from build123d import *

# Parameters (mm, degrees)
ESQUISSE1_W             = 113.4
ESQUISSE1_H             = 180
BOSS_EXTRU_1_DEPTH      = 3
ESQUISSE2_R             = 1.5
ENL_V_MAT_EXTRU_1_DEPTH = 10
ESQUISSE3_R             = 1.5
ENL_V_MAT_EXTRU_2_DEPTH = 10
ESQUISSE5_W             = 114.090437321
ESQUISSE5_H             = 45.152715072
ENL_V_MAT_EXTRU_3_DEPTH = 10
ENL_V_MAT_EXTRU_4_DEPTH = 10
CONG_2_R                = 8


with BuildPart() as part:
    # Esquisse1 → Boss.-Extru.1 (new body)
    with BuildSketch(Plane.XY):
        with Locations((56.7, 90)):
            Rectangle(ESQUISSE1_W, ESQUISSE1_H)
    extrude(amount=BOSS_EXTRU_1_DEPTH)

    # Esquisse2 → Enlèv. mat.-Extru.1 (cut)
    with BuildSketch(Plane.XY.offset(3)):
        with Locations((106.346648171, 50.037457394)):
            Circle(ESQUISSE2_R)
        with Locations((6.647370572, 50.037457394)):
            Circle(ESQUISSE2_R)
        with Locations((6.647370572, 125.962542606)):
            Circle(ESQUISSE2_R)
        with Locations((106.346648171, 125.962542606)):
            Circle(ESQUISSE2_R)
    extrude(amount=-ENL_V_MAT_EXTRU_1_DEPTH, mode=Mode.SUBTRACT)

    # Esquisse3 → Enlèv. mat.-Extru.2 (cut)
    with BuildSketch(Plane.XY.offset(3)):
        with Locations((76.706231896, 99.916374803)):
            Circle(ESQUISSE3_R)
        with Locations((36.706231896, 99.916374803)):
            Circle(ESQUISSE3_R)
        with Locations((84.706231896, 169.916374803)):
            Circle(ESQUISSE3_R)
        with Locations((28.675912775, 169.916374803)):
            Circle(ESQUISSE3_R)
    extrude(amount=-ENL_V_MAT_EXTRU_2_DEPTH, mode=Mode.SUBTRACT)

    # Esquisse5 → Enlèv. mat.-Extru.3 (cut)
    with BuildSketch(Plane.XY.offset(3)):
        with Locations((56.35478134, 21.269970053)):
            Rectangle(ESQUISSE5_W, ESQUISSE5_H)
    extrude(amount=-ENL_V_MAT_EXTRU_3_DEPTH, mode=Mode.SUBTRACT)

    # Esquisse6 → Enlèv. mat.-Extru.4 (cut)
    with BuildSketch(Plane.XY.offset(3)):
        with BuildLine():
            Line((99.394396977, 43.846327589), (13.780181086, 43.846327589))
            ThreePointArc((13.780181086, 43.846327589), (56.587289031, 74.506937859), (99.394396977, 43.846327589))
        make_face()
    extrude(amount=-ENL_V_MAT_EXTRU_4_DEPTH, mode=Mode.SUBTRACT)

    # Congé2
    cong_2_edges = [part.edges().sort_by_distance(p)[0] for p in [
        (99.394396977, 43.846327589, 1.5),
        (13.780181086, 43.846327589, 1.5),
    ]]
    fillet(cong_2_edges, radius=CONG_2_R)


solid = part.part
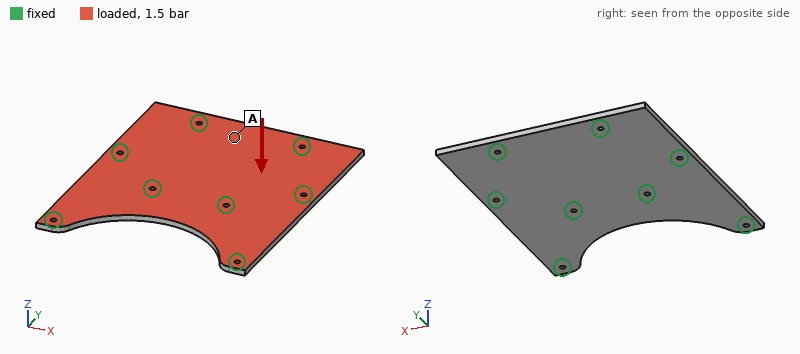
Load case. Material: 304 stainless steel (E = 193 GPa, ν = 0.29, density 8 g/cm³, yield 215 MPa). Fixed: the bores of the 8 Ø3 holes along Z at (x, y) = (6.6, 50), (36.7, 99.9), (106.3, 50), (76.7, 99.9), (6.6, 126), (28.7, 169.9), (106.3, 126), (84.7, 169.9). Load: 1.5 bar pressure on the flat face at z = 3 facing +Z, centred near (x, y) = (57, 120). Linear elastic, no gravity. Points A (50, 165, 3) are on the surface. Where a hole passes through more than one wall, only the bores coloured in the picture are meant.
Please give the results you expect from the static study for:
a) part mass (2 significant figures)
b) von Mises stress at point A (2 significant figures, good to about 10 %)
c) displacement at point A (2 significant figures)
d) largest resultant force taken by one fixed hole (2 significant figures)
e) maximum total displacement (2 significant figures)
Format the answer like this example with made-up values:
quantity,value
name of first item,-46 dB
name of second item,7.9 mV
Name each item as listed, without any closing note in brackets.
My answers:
quantity,value
part mass,320 g
von Mises stress at point A,13 MPa
displacement at point A,14 µm
largest resultant force taken by one fixed hole,360 N
maximum total displacement,24 µm
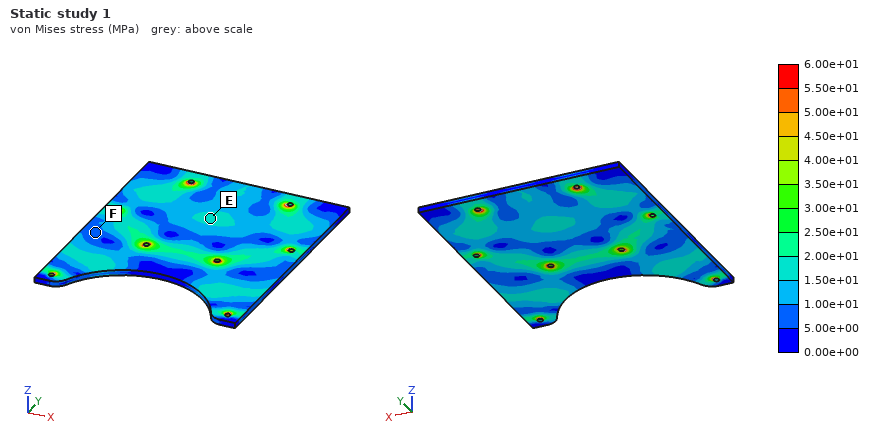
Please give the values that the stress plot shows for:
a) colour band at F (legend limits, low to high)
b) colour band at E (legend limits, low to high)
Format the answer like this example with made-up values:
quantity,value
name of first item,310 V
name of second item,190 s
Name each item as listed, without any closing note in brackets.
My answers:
quantity,value
colour band at F,5.00e+00 to 1.00e+01 MPa
colour band at E,1.50e+01 to 2.00e+01 MPa
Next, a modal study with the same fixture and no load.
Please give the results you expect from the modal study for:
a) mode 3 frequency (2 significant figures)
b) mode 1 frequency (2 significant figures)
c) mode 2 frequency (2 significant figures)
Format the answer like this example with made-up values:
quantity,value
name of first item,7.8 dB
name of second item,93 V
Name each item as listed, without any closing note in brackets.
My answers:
quantity,value
mode 3 frequency,3300 Hz
mode 1 frequency,2800 Hz
mode 2 frequency,3300 Hz
